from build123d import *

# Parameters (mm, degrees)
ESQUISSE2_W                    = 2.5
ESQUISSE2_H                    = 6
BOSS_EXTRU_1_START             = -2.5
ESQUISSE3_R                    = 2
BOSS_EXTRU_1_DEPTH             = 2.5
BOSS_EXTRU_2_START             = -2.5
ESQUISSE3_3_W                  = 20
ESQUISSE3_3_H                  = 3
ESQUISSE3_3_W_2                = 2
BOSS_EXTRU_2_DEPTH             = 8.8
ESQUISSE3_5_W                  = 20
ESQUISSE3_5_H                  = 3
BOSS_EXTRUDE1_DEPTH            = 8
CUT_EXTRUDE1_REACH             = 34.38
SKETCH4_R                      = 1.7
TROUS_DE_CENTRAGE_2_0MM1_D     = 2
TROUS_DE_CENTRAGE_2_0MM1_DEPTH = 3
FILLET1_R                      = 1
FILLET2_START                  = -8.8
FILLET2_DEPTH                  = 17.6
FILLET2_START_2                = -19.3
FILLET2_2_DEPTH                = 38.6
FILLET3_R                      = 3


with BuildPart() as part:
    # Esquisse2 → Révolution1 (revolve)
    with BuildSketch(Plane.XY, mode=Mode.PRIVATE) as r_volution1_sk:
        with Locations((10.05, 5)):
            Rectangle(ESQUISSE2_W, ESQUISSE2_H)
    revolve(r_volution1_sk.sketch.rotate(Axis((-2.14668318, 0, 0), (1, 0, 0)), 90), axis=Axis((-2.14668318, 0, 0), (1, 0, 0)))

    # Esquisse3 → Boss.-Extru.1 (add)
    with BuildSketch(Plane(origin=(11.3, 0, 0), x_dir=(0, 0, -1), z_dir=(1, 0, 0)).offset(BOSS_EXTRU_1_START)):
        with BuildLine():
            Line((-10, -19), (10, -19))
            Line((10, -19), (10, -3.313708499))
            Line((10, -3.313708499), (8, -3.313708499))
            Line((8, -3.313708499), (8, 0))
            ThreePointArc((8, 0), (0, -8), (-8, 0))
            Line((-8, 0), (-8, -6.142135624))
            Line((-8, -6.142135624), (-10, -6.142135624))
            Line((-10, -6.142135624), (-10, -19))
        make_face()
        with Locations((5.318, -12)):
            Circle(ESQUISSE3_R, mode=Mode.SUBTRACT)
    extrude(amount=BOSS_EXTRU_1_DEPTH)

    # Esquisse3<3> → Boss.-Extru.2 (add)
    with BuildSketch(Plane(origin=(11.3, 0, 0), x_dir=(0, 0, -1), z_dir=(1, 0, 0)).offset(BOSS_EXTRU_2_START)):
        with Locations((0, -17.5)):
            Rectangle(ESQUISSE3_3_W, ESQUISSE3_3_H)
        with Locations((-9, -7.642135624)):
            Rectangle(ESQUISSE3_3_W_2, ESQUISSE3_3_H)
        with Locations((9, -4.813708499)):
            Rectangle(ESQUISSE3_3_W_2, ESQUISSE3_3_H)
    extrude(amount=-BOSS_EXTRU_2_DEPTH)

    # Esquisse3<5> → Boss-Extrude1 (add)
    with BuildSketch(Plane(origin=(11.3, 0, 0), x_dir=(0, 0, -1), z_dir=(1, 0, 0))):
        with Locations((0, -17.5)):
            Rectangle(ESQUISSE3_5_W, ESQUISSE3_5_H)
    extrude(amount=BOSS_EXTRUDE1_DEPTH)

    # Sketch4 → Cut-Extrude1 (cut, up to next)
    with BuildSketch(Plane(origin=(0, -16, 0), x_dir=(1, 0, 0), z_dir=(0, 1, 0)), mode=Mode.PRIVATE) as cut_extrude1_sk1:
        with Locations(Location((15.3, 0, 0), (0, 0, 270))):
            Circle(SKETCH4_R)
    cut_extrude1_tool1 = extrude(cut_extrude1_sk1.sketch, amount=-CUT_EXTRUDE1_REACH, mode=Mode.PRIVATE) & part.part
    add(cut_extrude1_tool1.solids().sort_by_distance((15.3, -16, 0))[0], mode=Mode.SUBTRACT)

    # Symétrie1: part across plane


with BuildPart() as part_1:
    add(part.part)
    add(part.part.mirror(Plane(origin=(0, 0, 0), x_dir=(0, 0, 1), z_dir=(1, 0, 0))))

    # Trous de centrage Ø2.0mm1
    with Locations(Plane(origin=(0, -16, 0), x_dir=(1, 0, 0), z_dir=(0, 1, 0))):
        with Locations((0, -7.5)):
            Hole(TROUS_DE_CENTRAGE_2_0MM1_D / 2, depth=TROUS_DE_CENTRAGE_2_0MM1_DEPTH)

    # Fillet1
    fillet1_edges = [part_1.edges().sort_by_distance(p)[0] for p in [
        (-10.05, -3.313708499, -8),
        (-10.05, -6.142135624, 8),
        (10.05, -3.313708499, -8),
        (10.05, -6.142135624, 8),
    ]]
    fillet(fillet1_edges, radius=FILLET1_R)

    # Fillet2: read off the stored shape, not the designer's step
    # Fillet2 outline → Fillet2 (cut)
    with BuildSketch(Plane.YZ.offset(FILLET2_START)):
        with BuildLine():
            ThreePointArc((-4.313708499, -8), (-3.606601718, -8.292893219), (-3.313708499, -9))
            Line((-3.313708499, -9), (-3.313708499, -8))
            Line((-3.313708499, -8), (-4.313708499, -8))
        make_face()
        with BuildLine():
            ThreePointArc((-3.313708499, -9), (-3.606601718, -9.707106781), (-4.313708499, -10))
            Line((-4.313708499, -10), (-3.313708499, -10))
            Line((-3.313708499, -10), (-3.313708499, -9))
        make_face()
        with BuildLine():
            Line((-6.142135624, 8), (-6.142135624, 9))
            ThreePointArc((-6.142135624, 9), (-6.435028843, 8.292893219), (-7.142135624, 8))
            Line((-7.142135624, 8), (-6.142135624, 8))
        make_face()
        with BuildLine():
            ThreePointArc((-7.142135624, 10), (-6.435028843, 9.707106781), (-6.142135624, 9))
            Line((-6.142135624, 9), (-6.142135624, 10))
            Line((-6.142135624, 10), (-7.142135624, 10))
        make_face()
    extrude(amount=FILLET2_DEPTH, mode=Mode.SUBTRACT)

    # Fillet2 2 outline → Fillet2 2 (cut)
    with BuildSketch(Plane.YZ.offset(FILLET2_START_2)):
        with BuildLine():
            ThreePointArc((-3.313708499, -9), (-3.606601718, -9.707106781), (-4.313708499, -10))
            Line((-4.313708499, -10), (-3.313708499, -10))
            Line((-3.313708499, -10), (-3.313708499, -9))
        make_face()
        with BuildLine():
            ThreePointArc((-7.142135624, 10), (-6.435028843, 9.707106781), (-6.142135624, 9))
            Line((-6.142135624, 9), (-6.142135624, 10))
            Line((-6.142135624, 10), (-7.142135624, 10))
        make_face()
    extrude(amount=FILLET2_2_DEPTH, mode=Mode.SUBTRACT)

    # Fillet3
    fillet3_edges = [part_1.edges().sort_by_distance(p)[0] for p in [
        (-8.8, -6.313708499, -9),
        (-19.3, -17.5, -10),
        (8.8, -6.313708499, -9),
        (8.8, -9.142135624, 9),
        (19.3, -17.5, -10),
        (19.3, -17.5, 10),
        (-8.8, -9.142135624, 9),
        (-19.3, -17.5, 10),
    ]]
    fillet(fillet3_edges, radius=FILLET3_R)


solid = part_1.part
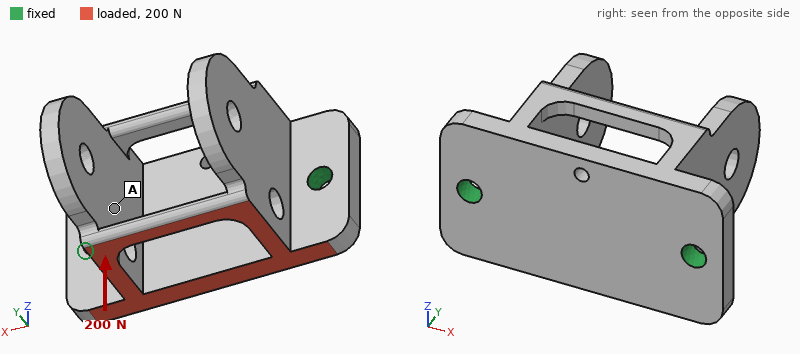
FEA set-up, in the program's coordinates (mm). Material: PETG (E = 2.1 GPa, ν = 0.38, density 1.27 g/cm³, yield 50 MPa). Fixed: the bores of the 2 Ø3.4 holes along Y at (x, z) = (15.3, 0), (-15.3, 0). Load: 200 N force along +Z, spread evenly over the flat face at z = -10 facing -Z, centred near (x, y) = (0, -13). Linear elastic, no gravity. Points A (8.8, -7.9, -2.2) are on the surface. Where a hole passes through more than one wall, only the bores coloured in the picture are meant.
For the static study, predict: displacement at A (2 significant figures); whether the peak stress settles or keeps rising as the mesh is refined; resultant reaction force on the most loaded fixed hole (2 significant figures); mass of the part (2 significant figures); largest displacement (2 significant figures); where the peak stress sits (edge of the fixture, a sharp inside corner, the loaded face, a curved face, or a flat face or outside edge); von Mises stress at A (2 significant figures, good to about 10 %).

0.19 mm
keeps rising
100 N
5.5 g
0.53 mm
edge of the fixture
4.2 MPa
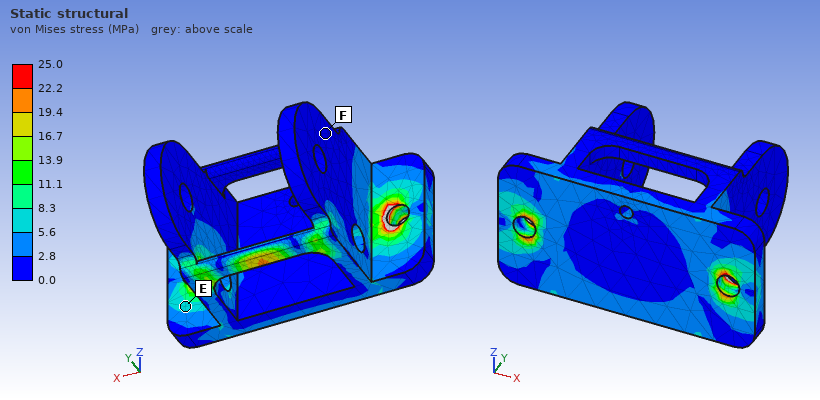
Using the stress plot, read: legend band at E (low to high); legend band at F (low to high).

5.6 to 8.3 MPa
0.0 to 2.8 MPa
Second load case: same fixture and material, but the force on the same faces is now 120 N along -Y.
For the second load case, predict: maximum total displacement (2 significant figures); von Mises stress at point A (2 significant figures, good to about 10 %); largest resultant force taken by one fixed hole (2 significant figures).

0.53 mm
3.1 MPa
61 N
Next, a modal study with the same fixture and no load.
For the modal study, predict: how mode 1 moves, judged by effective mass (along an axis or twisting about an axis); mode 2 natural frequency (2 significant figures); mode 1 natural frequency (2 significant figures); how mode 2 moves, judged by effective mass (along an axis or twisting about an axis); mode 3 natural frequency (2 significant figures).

along X
1500 Hz
1300 Hz
along Z
1800 Hz
